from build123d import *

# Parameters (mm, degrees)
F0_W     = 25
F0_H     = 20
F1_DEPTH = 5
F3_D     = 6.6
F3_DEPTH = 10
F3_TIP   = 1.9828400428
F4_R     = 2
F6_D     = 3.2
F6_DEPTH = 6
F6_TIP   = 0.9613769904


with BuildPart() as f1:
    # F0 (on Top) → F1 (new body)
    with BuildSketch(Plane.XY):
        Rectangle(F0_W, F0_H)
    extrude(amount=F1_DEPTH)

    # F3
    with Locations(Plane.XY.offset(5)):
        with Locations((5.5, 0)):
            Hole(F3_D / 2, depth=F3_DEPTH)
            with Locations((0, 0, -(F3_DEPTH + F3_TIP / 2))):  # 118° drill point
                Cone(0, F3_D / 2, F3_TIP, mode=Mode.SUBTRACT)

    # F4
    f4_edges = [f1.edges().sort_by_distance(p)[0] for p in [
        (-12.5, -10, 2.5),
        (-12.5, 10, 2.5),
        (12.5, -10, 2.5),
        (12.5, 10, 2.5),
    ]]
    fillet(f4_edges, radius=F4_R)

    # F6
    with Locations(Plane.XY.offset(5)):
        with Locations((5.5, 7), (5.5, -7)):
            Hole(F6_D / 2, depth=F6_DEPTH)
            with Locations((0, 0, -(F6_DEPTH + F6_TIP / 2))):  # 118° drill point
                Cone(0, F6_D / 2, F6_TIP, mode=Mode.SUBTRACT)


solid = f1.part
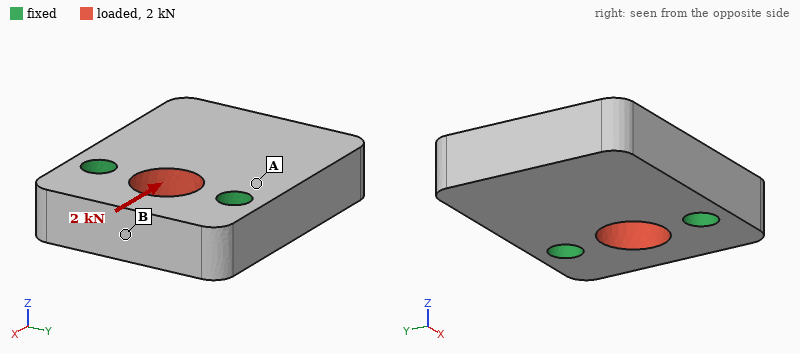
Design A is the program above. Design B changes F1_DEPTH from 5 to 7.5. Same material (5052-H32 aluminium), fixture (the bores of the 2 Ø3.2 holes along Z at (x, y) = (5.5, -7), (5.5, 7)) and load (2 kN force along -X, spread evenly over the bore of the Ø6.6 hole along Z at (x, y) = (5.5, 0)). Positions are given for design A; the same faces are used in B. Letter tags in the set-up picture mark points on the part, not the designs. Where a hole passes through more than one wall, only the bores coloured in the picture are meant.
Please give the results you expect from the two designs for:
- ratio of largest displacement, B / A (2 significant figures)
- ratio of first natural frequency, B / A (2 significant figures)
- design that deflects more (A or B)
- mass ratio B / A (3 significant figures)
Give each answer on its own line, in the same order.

0.67
1.4
A
1.50
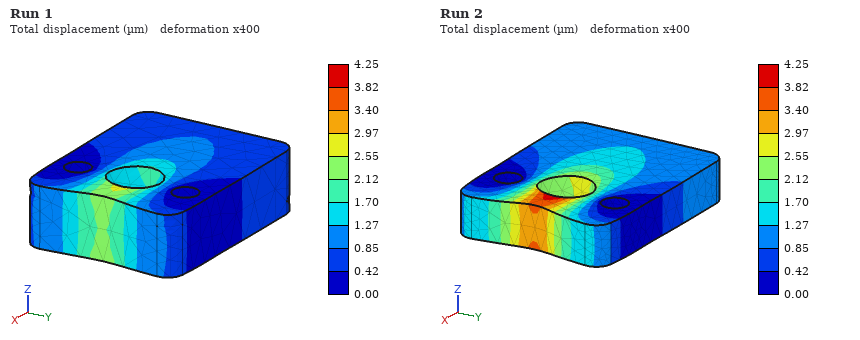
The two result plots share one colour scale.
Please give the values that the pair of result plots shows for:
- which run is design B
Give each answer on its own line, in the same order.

Run 1
